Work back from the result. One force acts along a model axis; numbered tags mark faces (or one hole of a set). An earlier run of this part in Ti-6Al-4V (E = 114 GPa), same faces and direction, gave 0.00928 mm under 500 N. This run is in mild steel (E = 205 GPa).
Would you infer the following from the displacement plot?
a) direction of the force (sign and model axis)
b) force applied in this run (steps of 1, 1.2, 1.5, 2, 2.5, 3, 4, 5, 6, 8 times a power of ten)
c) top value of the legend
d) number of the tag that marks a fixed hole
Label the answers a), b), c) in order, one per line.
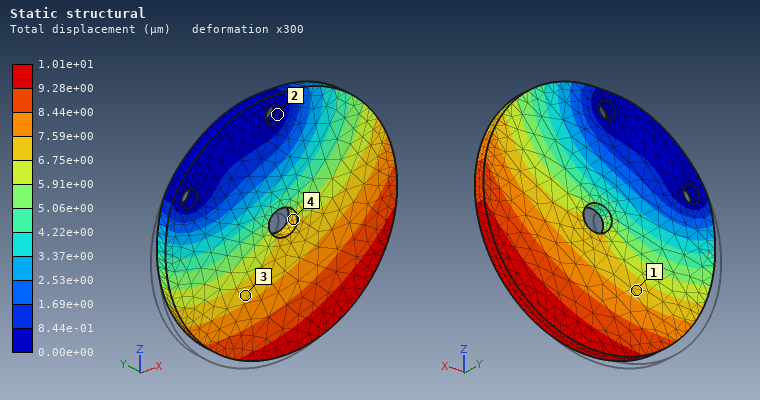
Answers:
a) +X
b) 1 kN
c) 1.01e+01 µm
d) 2
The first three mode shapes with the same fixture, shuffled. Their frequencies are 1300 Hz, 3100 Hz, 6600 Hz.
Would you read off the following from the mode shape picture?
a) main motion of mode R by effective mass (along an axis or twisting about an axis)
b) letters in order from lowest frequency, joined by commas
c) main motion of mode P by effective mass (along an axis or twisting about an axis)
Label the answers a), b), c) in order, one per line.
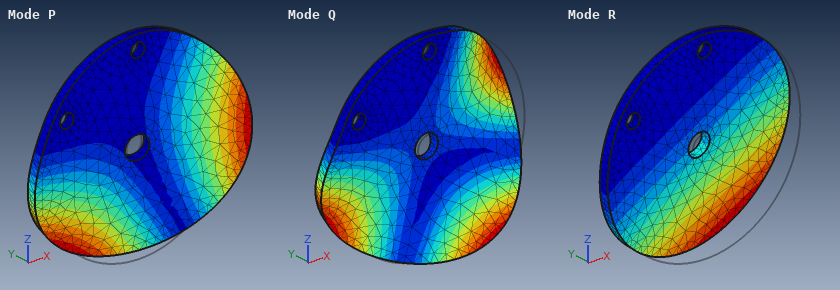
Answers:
a) along Y
b) R, P, Q
c) twisting about Z
